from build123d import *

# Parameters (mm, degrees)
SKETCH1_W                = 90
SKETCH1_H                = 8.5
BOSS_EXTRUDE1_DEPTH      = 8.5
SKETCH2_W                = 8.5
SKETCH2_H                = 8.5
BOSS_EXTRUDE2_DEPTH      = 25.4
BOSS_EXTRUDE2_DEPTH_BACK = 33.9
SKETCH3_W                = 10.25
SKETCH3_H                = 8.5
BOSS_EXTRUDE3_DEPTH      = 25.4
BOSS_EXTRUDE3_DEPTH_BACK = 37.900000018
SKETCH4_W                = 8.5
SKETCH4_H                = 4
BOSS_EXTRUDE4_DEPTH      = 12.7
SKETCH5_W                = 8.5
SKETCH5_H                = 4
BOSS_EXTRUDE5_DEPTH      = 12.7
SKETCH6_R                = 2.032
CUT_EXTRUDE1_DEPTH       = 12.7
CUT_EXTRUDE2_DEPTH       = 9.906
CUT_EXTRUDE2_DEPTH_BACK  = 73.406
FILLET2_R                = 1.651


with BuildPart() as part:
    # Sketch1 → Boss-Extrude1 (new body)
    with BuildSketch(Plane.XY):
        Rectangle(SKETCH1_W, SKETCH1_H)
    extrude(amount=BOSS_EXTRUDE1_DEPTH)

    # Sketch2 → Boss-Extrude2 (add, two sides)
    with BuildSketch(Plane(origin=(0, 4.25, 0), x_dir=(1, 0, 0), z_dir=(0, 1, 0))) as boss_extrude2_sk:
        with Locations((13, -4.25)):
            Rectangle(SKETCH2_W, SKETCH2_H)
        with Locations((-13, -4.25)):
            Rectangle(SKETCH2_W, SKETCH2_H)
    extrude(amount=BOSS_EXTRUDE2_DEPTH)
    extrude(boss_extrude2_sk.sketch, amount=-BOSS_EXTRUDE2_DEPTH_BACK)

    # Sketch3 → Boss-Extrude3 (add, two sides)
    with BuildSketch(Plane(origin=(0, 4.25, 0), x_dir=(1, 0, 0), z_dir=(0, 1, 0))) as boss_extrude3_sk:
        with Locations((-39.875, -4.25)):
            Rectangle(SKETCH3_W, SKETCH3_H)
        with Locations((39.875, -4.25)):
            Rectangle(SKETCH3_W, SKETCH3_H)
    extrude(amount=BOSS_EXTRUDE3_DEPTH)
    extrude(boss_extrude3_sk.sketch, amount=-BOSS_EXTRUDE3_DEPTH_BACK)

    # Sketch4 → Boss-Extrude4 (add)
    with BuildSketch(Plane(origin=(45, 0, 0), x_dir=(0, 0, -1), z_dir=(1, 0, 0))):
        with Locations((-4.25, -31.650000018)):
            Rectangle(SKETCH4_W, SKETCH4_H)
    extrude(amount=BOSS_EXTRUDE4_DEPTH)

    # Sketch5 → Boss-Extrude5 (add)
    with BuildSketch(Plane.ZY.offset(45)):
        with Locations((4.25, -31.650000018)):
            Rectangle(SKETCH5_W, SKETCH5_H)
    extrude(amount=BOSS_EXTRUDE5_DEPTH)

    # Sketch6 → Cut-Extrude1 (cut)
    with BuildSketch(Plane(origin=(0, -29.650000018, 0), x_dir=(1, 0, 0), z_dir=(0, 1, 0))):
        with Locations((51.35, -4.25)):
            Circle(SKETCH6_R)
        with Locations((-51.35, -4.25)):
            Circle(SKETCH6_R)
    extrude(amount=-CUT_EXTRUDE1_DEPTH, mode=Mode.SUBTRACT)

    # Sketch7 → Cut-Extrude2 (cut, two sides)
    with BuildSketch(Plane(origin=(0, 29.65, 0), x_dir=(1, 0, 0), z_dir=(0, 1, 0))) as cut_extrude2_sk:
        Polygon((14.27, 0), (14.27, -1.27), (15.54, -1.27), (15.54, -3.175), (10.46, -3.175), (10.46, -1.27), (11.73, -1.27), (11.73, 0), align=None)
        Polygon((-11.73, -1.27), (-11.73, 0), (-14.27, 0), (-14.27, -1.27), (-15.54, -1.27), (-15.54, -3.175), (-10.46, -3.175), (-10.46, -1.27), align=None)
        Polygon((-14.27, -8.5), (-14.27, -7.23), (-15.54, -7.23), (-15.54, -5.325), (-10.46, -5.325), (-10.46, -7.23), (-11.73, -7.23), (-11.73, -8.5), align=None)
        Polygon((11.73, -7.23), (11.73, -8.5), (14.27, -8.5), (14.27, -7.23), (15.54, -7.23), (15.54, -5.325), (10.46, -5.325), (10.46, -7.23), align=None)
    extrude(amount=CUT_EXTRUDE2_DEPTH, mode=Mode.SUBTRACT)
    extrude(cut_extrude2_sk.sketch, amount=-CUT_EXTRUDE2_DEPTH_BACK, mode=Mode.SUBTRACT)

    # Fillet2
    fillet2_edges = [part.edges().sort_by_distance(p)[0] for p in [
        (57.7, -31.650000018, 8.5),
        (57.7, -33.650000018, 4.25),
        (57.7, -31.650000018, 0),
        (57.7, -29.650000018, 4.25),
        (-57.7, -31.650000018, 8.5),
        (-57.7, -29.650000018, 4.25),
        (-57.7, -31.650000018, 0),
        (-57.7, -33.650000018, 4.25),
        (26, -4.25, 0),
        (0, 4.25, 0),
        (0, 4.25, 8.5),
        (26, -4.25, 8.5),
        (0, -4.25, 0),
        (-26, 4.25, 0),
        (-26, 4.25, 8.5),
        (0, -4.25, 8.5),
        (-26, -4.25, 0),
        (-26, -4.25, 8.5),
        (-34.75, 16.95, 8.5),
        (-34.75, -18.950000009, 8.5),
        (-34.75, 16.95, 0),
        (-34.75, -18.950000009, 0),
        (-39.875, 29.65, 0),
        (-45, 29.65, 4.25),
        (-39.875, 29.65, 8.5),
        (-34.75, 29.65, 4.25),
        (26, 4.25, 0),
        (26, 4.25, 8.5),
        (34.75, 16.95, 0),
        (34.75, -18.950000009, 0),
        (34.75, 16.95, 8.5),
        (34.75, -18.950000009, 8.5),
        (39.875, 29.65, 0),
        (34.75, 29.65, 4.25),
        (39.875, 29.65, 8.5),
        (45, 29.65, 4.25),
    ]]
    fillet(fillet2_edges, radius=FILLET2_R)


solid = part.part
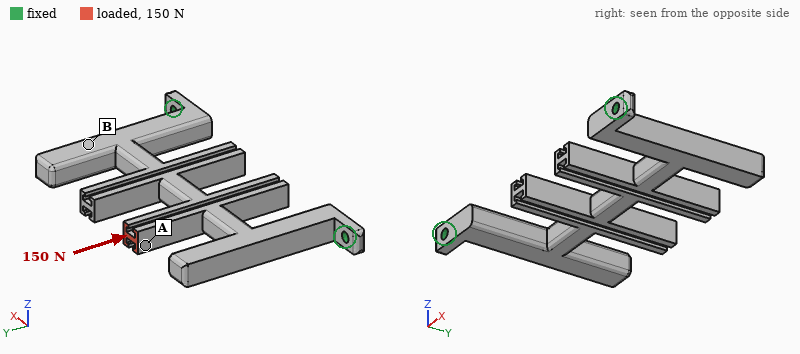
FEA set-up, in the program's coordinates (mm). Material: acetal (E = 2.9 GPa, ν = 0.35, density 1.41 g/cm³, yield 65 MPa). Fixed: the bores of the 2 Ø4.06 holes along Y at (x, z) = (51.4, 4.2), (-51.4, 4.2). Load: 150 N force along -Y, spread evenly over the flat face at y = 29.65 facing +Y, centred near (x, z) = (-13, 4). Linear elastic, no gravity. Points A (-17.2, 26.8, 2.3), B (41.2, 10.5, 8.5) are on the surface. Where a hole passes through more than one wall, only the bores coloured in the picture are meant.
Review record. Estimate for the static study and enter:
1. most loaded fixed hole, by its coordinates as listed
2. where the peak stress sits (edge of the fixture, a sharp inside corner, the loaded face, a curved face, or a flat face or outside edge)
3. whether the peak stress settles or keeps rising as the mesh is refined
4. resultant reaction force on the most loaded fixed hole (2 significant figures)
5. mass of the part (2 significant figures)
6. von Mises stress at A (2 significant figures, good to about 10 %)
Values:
(-51.4, 4.2)
edge of the fixture
keeps rising
110 N
29 g
3.2 MPa
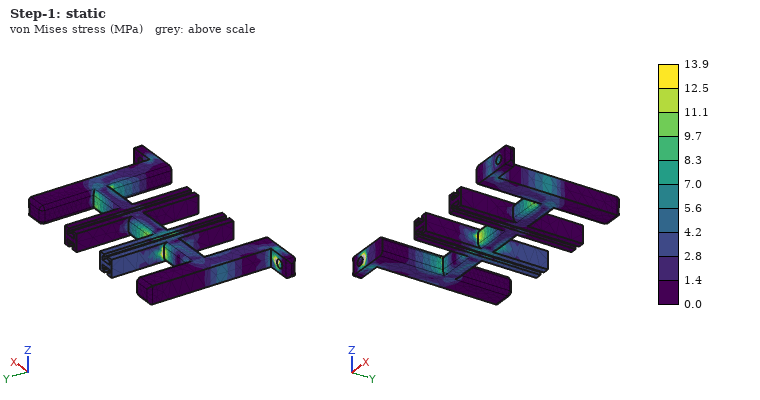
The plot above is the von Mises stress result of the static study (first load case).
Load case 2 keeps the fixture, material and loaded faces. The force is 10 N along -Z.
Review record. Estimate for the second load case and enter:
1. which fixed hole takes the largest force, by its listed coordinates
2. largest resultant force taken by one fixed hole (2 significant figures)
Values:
(-51.4, 4.2)
6.5 N
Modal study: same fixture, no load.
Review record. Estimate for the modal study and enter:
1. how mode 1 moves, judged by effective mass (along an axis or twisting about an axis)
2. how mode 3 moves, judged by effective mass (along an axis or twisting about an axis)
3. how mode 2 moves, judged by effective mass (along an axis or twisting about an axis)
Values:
along Z
along X
twisting about Y
